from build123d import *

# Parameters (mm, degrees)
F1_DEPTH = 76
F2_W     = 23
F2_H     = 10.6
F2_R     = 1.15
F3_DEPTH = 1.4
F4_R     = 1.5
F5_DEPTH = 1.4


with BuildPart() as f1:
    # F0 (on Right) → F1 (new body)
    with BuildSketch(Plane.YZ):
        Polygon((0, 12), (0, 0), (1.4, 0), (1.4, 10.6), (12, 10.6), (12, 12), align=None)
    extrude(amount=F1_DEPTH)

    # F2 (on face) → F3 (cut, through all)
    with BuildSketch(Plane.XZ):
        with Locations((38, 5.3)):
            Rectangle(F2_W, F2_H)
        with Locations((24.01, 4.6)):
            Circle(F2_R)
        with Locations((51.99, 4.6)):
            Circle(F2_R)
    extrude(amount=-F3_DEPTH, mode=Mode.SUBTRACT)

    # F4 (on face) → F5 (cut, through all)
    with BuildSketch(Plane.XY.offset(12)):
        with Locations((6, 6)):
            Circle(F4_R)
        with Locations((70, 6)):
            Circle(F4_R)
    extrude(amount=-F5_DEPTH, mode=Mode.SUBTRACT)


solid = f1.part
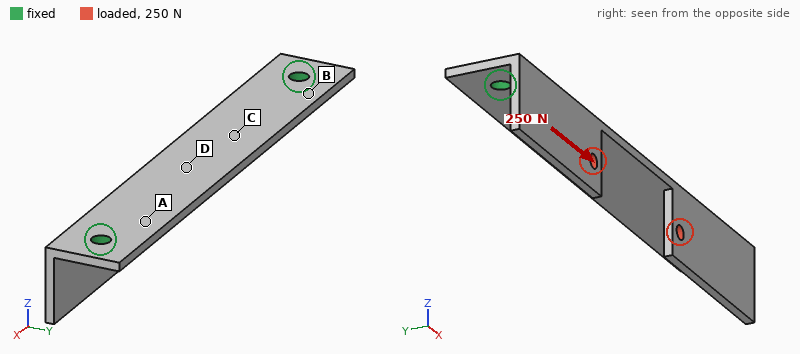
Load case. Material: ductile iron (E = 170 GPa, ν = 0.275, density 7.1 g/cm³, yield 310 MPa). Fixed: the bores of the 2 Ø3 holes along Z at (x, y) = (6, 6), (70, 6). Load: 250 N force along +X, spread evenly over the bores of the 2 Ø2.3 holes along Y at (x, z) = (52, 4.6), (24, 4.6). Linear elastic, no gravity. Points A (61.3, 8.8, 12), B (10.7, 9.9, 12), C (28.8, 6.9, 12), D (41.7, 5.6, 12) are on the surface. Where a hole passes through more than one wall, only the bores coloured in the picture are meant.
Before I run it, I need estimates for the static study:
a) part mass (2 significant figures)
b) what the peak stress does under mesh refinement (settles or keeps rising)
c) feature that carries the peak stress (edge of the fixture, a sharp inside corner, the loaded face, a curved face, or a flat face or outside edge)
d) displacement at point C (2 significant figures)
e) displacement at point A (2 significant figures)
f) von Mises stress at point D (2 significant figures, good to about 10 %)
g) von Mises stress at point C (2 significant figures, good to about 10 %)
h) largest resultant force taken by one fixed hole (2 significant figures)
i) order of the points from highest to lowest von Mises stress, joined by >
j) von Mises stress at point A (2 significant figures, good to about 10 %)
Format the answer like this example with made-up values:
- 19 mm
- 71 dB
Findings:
- 14 g
- keeps rising
- edge of the fixture
- 15 µm
- 5.7 µm
- 28 MPa
- 36 MPa
- 130 N
- C > D > B > A
- 6.9 MPa
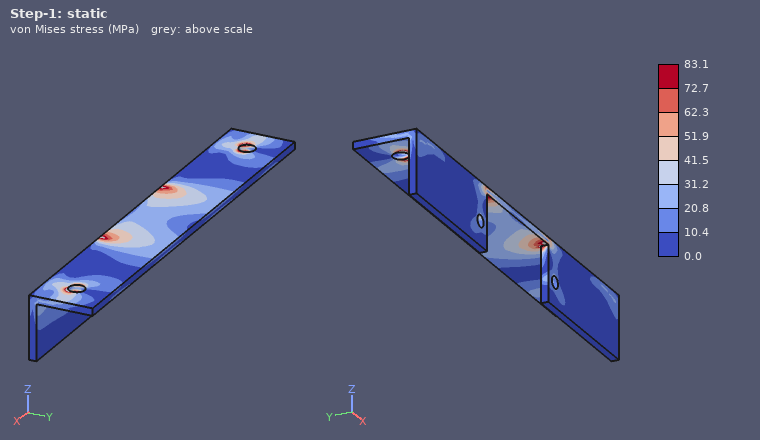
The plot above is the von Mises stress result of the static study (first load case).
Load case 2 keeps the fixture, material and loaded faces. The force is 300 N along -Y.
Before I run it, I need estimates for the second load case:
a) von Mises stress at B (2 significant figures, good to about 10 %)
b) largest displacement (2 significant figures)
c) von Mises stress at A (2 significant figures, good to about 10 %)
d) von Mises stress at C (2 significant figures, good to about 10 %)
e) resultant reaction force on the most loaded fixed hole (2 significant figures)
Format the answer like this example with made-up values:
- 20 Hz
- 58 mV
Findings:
- 88 MPa
- 0.24 mm
- 90 MPa
- 38 MPa
- 150 N
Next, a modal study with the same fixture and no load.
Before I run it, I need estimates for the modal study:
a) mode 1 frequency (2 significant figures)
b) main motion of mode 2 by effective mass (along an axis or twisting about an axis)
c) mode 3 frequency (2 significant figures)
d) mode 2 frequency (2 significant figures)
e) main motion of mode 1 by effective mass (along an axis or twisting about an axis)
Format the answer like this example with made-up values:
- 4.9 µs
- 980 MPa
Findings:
- 2300 Hz
- along Y
- 4300 Hz
- 3700 Hz
- along Z
